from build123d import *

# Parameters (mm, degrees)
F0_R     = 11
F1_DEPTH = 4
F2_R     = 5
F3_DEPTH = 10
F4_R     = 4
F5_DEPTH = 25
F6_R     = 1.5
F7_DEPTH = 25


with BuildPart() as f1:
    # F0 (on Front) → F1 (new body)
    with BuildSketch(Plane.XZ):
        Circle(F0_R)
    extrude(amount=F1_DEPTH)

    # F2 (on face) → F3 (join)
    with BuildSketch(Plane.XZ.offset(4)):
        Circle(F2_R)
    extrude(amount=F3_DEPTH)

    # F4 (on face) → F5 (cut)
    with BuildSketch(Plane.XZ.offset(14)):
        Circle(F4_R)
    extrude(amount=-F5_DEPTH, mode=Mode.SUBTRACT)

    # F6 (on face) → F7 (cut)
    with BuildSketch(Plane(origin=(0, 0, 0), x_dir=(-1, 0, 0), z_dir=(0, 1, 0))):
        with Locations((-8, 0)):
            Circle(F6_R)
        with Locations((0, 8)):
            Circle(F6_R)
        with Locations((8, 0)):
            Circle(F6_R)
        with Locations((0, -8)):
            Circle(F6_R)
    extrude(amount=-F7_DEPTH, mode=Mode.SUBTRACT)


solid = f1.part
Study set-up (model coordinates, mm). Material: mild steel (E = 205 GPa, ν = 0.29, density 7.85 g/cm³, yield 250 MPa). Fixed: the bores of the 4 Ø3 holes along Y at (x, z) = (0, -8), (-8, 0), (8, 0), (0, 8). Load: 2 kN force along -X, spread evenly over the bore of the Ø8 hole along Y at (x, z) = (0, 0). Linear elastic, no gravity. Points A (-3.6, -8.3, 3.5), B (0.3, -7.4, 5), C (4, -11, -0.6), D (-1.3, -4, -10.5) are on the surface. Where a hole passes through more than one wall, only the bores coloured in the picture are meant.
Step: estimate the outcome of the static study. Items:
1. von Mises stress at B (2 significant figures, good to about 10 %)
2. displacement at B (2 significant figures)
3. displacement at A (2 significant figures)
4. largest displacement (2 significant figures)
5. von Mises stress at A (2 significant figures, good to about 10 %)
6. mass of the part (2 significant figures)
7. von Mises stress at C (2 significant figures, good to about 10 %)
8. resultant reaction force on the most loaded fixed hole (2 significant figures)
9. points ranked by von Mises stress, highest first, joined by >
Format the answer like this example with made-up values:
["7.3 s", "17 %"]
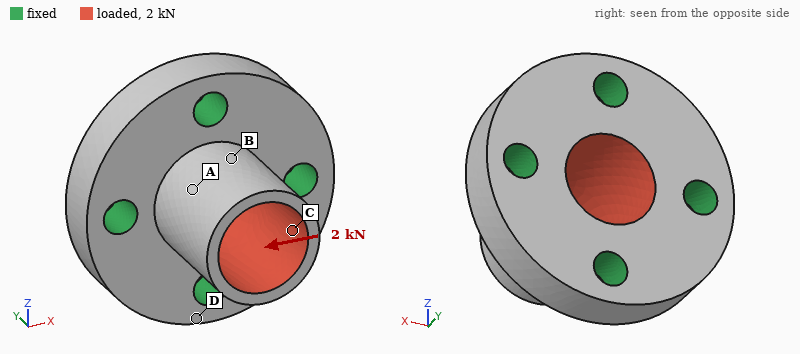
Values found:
["99 MPa", "5.5 µm", "7.7 µm", "14 µm", "69 MPa", "12 g", "39 MPa", "900 N", "B > A > C > D"]
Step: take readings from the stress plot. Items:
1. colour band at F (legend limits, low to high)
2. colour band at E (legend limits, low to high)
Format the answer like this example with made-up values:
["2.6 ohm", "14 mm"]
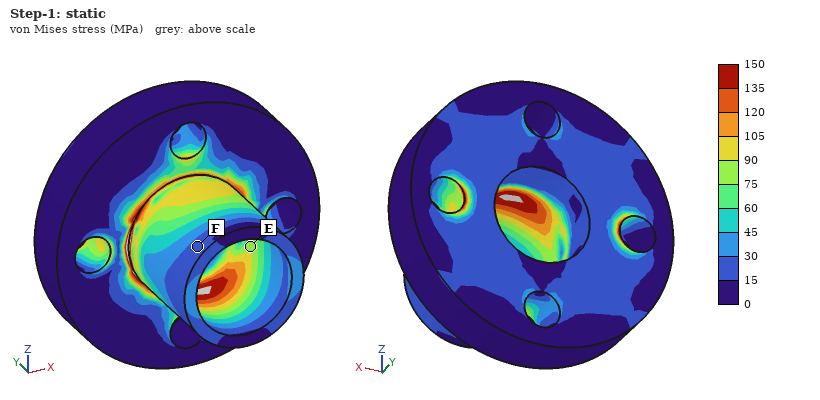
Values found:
["15 to 30 MPa", "75 to 90 MPa"]
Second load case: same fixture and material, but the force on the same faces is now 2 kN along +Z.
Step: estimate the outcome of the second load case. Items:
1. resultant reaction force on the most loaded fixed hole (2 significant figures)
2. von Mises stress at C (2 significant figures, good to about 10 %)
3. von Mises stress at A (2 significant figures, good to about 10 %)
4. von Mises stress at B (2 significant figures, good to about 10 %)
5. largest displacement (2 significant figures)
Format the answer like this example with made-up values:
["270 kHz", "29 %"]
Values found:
["900 N", "57 MPa", "71 MPa", "42 MPa", "14 µm"]
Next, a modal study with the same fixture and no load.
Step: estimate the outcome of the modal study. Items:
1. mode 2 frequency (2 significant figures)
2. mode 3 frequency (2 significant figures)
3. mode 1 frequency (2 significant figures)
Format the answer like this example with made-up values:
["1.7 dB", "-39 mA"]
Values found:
["40 kHz", "40 kHz", "40 kHz"]
